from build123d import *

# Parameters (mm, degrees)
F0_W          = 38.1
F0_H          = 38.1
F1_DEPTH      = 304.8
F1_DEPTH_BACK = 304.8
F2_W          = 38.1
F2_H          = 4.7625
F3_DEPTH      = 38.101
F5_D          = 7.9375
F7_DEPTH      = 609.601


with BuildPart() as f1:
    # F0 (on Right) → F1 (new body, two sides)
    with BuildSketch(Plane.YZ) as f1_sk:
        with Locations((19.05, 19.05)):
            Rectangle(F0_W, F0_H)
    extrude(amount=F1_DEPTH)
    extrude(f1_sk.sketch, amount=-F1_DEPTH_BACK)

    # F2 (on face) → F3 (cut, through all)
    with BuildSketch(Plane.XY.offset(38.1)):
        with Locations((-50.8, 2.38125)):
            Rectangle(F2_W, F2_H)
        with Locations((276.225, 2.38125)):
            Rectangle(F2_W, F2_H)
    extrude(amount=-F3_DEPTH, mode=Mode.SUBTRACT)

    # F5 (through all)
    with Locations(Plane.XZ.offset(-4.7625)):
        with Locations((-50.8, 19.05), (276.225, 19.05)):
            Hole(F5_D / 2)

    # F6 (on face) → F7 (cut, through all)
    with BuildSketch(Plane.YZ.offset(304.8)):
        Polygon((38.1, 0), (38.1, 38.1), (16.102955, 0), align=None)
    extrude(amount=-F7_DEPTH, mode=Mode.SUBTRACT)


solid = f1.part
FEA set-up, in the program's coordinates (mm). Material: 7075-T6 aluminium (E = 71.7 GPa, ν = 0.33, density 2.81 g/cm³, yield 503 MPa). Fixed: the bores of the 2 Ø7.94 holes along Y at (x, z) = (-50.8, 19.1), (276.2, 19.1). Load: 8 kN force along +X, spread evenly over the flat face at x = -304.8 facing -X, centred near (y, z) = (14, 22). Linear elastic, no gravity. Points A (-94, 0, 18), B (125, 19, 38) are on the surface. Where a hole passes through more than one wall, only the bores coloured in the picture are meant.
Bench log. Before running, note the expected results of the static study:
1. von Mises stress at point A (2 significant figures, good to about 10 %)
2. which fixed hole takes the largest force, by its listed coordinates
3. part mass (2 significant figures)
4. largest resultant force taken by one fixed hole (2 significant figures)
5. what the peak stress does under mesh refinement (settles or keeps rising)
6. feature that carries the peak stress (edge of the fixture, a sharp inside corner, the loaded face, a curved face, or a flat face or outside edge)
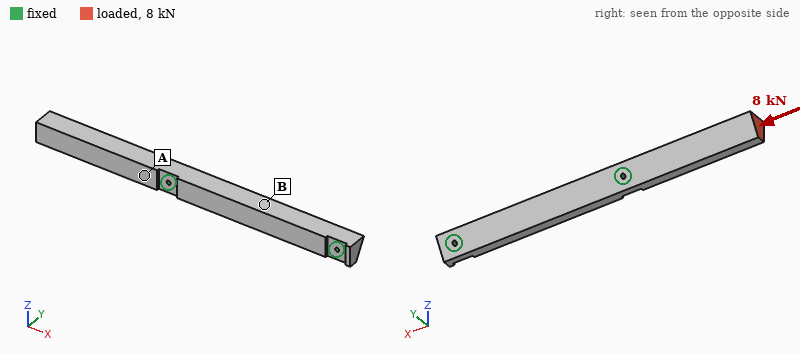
7.5 MPa
(-50.8, 19.1)
1.7 kg
7.7 kN
keeps rising
edge of the fixture
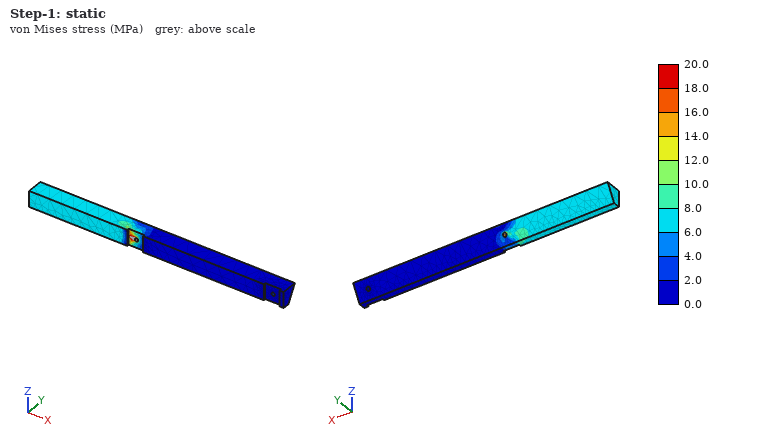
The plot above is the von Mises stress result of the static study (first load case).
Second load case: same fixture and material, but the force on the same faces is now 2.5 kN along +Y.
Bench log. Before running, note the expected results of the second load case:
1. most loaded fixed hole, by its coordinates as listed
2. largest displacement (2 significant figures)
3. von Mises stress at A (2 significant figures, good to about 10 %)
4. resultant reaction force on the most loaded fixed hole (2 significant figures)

(-50.8, 19.1)
3.5 mm
92 MPa
2.8 kN
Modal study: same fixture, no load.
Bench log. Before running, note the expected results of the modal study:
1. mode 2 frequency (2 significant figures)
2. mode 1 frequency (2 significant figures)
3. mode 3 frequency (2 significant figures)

390 Hz
290 Hz
1000 Hz
